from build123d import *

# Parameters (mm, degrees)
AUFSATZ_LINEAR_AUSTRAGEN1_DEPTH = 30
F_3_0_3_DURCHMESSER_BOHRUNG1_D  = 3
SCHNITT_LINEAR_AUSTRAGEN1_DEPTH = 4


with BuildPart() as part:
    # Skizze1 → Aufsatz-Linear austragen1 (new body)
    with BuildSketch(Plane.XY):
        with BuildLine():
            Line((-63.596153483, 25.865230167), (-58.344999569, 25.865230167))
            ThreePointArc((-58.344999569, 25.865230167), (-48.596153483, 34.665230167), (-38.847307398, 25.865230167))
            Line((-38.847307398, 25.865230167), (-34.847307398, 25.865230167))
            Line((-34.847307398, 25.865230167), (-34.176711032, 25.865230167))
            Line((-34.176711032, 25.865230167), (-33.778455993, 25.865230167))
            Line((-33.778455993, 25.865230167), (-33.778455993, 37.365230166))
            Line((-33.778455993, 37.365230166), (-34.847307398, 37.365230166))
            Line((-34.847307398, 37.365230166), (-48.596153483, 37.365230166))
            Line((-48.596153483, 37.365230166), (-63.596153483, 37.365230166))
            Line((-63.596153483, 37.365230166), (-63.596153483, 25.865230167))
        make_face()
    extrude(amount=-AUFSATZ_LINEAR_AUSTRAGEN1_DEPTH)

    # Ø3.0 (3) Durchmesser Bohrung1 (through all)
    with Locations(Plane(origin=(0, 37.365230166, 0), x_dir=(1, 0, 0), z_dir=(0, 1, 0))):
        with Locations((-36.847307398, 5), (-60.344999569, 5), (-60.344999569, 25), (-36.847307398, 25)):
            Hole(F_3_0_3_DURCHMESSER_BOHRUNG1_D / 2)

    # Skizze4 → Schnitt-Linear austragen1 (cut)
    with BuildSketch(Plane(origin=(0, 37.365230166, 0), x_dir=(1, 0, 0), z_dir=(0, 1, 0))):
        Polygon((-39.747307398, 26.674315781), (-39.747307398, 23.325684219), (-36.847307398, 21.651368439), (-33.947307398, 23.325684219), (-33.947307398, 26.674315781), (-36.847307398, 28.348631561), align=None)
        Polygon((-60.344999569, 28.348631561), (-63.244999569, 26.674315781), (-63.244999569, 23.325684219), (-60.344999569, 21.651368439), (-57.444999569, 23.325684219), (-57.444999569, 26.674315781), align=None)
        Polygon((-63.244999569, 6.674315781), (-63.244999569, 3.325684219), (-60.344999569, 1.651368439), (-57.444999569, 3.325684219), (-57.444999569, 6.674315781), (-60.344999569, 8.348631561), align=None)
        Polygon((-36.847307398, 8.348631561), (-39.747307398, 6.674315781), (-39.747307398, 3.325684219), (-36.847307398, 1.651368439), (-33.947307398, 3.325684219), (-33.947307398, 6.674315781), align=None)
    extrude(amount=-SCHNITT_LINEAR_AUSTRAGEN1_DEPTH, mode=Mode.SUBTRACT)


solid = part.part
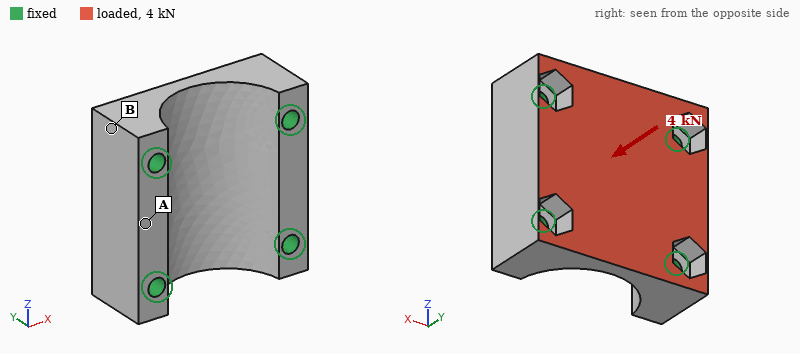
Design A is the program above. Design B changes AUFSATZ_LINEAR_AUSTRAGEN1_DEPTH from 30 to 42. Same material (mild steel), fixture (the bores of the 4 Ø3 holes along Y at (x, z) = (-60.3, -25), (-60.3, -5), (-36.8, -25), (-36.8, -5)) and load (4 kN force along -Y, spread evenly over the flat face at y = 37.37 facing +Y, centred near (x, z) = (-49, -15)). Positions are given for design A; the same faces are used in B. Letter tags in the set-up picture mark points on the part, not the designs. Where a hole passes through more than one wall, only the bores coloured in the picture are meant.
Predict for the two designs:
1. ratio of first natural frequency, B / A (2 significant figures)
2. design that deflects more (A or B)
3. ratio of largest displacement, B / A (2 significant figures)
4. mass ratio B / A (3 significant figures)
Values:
0.41
B
3.0
1.45
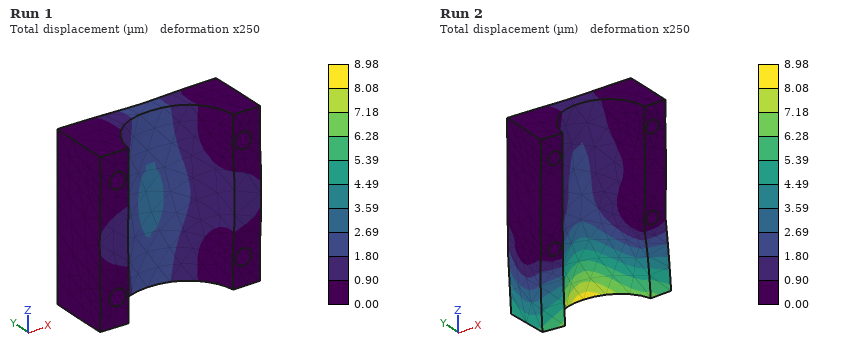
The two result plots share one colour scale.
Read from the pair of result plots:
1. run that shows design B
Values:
Run 2
